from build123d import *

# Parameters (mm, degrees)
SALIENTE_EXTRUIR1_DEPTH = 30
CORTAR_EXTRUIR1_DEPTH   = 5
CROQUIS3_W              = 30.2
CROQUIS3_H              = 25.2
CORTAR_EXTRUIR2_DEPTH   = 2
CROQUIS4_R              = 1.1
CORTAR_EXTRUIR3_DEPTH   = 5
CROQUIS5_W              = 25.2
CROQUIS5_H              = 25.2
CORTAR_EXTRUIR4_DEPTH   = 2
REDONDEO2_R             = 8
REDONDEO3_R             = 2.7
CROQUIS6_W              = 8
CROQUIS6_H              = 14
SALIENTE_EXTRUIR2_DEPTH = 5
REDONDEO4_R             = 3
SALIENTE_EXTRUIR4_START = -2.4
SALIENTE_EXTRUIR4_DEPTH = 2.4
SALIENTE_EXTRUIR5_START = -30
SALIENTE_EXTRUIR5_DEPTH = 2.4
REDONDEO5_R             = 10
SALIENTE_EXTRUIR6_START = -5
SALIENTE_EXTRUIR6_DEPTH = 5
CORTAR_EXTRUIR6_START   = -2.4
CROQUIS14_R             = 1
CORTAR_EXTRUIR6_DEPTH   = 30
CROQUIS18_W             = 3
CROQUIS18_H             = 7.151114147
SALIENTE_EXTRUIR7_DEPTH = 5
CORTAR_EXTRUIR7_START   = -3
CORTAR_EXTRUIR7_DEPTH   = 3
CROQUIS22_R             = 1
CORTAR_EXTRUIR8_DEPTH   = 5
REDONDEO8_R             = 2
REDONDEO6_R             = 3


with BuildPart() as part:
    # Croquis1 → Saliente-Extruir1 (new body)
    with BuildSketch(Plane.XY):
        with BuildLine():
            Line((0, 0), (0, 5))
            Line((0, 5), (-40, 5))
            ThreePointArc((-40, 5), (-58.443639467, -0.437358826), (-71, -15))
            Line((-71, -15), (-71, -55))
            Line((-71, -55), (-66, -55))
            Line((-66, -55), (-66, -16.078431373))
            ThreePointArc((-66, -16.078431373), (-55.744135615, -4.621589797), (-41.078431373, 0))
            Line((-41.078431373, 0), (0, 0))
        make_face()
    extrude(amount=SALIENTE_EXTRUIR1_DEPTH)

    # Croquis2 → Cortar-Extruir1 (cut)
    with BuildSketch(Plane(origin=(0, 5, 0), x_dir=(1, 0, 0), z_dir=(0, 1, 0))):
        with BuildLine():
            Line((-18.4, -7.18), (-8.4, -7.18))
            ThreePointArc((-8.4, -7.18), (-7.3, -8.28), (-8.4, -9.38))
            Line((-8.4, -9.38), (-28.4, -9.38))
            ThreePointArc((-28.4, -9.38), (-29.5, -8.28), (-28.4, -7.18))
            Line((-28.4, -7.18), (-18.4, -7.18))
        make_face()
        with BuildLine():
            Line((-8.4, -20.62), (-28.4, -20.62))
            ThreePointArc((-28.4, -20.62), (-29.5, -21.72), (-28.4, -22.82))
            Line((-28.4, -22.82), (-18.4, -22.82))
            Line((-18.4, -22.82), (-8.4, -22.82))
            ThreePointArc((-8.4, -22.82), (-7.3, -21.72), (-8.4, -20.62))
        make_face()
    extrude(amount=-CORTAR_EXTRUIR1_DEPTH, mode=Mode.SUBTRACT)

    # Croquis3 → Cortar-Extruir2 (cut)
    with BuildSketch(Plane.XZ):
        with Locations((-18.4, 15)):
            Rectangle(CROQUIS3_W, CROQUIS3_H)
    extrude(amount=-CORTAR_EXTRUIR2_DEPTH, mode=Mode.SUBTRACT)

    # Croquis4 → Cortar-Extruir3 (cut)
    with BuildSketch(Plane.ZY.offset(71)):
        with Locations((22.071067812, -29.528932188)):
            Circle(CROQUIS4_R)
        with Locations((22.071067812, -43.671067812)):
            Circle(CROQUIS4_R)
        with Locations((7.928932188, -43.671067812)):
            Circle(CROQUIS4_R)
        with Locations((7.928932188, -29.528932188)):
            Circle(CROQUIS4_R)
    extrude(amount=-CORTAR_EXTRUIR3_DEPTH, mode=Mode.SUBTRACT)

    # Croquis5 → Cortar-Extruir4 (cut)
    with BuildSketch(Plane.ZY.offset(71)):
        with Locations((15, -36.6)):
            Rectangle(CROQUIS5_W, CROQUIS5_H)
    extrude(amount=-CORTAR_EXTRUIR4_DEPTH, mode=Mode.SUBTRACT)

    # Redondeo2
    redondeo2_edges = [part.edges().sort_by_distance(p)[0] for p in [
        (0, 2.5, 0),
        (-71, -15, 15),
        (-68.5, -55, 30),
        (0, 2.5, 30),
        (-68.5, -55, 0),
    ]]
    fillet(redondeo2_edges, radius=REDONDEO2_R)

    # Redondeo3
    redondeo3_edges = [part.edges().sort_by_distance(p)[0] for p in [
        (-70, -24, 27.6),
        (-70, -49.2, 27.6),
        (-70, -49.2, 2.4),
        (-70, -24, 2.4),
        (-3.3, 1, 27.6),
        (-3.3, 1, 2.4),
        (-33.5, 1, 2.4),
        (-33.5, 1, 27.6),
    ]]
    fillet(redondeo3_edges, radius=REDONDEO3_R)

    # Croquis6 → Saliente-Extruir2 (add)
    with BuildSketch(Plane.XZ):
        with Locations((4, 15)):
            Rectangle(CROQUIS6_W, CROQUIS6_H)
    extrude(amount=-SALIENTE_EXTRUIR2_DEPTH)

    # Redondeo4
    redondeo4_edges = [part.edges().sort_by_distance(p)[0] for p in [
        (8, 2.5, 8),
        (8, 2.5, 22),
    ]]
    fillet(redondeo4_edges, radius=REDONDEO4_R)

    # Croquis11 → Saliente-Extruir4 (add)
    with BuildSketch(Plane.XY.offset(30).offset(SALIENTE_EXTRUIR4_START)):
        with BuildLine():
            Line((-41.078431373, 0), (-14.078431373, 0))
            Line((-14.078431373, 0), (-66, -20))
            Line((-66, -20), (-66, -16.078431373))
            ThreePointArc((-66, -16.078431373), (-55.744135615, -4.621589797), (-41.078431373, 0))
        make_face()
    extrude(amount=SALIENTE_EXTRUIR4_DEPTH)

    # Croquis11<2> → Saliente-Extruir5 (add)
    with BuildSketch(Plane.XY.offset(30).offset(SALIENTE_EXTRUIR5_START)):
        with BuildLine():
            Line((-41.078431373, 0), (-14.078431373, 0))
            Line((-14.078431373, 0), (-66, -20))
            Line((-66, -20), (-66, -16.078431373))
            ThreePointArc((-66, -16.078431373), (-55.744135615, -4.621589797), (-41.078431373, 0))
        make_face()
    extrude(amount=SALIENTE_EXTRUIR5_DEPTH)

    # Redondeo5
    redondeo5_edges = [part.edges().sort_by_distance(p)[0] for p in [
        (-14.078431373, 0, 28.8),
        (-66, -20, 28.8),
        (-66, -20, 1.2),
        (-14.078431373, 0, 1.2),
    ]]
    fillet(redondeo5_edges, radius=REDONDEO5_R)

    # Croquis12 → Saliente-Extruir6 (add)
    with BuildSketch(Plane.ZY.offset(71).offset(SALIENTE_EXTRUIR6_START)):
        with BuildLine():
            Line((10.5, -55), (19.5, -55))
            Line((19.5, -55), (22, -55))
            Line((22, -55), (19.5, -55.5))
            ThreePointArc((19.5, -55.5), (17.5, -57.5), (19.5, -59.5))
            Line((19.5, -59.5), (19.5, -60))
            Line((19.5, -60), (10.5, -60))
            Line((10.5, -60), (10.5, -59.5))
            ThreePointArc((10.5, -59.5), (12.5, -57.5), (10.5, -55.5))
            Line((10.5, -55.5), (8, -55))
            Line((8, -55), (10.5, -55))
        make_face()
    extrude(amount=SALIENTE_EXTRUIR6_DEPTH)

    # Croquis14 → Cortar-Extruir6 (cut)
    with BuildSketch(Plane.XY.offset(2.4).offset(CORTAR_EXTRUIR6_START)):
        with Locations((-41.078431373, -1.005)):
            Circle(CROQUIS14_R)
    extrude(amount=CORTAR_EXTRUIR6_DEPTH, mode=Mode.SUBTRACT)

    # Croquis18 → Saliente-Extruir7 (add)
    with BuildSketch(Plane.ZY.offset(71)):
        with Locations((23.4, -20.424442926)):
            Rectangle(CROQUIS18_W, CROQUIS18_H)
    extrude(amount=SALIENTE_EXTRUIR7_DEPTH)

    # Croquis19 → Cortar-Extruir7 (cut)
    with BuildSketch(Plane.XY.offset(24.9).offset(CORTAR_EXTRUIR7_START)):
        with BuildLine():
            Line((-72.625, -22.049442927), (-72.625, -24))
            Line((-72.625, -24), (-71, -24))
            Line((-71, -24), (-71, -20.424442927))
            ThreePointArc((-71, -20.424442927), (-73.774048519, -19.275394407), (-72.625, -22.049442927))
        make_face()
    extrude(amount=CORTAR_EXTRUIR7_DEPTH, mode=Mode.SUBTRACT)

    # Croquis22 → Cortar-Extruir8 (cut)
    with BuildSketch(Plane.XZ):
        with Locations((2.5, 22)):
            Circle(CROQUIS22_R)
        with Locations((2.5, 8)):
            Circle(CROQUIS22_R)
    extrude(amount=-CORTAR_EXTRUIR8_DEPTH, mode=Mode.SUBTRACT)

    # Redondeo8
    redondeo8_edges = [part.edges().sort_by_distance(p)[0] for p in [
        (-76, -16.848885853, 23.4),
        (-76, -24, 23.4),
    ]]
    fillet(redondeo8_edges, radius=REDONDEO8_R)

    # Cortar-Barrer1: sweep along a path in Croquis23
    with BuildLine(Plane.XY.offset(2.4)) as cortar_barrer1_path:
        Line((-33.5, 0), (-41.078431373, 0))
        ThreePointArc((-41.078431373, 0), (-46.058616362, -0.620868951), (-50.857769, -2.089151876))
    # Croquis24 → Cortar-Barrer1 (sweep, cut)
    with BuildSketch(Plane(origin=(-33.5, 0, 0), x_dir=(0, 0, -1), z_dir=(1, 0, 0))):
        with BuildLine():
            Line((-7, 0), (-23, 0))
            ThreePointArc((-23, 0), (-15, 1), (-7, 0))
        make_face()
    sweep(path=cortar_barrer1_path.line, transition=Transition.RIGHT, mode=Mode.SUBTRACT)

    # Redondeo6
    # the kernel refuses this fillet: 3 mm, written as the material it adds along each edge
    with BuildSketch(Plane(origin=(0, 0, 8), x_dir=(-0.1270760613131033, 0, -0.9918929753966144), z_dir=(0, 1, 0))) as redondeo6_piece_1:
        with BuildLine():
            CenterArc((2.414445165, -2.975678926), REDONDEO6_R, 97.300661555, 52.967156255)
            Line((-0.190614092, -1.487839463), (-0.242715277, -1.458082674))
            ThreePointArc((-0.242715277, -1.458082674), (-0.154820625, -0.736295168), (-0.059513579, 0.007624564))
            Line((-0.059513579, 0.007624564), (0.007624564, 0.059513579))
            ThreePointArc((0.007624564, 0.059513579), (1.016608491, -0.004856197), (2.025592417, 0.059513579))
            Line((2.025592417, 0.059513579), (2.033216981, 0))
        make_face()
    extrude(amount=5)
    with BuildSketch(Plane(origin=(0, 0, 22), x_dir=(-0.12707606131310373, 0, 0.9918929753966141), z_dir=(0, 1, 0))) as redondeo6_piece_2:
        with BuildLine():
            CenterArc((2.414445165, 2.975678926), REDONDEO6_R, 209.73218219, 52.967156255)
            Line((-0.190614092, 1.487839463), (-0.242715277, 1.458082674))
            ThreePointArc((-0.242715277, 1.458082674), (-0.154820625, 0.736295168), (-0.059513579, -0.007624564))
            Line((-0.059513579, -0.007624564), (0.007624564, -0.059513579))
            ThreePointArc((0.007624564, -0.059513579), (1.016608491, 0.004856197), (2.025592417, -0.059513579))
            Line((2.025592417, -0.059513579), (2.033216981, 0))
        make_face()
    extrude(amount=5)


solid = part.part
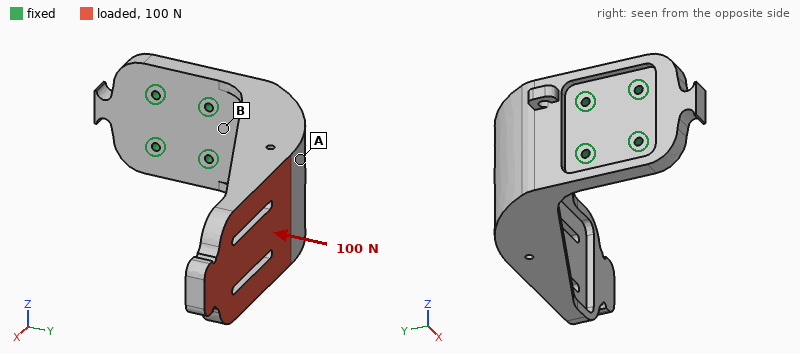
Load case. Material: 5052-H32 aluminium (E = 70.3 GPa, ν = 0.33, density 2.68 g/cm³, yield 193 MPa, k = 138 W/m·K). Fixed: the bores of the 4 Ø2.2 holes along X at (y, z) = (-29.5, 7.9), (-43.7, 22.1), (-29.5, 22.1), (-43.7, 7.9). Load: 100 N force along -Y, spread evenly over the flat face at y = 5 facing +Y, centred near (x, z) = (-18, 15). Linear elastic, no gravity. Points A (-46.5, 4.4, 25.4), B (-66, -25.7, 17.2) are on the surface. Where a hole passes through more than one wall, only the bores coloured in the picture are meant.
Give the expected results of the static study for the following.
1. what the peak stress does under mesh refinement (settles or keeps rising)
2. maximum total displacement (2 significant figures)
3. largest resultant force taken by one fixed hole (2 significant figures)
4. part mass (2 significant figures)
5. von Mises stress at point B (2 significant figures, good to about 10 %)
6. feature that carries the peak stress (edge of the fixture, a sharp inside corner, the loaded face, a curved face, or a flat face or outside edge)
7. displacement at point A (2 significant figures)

keeps rising
0.58 mm
150 N
44 g
60 MPa
edge of the fixture
0.23 mm
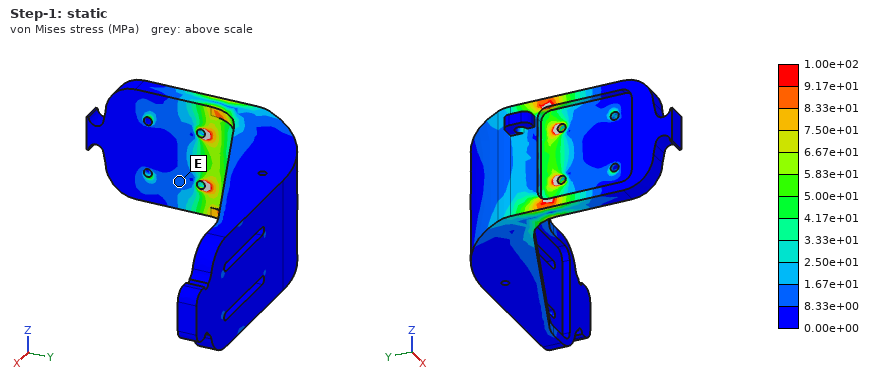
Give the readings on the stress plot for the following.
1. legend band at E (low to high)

8.33e+00 to 1.67e+01 MPa
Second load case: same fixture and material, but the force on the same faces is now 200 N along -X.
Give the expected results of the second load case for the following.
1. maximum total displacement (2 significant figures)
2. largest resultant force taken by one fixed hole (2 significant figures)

0.65 mm
260 N
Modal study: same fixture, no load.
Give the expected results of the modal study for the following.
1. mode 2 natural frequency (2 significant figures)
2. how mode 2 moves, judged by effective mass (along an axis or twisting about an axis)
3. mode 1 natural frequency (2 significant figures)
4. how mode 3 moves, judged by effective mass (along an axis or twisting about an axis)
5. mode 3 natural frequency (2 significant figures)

1000 Hz
along Z
580 Hz
along X
3200 Hz
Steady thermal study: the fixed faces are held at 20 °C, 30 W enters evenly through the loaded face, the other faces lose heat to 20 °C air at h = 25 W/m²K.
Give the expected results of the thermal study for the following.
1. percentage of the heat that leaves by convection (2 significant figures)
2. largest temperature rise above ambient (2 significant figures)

28 %
87 K
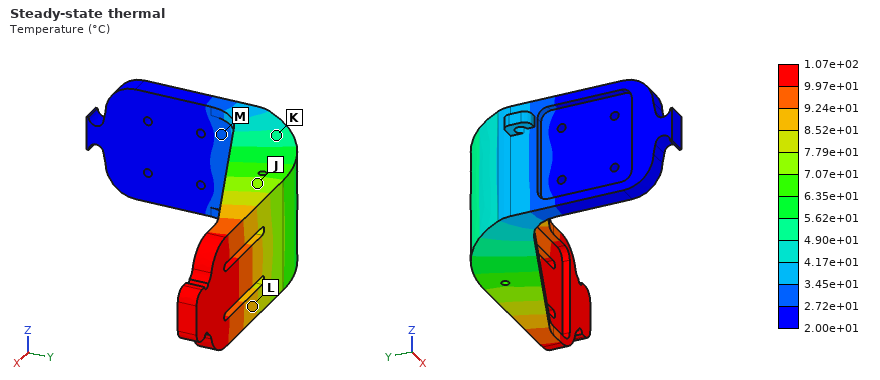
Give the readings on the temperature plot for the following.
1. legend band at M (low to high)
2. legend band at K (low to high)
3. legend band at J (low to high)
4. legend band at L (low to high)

2.72e+01 to 3.45e+01 °C
4.90e+01 to 5.62e+01 °C
7.07e+01 to 7.79e+01 °C
8.52e+01 to 9.24e+01 °C
